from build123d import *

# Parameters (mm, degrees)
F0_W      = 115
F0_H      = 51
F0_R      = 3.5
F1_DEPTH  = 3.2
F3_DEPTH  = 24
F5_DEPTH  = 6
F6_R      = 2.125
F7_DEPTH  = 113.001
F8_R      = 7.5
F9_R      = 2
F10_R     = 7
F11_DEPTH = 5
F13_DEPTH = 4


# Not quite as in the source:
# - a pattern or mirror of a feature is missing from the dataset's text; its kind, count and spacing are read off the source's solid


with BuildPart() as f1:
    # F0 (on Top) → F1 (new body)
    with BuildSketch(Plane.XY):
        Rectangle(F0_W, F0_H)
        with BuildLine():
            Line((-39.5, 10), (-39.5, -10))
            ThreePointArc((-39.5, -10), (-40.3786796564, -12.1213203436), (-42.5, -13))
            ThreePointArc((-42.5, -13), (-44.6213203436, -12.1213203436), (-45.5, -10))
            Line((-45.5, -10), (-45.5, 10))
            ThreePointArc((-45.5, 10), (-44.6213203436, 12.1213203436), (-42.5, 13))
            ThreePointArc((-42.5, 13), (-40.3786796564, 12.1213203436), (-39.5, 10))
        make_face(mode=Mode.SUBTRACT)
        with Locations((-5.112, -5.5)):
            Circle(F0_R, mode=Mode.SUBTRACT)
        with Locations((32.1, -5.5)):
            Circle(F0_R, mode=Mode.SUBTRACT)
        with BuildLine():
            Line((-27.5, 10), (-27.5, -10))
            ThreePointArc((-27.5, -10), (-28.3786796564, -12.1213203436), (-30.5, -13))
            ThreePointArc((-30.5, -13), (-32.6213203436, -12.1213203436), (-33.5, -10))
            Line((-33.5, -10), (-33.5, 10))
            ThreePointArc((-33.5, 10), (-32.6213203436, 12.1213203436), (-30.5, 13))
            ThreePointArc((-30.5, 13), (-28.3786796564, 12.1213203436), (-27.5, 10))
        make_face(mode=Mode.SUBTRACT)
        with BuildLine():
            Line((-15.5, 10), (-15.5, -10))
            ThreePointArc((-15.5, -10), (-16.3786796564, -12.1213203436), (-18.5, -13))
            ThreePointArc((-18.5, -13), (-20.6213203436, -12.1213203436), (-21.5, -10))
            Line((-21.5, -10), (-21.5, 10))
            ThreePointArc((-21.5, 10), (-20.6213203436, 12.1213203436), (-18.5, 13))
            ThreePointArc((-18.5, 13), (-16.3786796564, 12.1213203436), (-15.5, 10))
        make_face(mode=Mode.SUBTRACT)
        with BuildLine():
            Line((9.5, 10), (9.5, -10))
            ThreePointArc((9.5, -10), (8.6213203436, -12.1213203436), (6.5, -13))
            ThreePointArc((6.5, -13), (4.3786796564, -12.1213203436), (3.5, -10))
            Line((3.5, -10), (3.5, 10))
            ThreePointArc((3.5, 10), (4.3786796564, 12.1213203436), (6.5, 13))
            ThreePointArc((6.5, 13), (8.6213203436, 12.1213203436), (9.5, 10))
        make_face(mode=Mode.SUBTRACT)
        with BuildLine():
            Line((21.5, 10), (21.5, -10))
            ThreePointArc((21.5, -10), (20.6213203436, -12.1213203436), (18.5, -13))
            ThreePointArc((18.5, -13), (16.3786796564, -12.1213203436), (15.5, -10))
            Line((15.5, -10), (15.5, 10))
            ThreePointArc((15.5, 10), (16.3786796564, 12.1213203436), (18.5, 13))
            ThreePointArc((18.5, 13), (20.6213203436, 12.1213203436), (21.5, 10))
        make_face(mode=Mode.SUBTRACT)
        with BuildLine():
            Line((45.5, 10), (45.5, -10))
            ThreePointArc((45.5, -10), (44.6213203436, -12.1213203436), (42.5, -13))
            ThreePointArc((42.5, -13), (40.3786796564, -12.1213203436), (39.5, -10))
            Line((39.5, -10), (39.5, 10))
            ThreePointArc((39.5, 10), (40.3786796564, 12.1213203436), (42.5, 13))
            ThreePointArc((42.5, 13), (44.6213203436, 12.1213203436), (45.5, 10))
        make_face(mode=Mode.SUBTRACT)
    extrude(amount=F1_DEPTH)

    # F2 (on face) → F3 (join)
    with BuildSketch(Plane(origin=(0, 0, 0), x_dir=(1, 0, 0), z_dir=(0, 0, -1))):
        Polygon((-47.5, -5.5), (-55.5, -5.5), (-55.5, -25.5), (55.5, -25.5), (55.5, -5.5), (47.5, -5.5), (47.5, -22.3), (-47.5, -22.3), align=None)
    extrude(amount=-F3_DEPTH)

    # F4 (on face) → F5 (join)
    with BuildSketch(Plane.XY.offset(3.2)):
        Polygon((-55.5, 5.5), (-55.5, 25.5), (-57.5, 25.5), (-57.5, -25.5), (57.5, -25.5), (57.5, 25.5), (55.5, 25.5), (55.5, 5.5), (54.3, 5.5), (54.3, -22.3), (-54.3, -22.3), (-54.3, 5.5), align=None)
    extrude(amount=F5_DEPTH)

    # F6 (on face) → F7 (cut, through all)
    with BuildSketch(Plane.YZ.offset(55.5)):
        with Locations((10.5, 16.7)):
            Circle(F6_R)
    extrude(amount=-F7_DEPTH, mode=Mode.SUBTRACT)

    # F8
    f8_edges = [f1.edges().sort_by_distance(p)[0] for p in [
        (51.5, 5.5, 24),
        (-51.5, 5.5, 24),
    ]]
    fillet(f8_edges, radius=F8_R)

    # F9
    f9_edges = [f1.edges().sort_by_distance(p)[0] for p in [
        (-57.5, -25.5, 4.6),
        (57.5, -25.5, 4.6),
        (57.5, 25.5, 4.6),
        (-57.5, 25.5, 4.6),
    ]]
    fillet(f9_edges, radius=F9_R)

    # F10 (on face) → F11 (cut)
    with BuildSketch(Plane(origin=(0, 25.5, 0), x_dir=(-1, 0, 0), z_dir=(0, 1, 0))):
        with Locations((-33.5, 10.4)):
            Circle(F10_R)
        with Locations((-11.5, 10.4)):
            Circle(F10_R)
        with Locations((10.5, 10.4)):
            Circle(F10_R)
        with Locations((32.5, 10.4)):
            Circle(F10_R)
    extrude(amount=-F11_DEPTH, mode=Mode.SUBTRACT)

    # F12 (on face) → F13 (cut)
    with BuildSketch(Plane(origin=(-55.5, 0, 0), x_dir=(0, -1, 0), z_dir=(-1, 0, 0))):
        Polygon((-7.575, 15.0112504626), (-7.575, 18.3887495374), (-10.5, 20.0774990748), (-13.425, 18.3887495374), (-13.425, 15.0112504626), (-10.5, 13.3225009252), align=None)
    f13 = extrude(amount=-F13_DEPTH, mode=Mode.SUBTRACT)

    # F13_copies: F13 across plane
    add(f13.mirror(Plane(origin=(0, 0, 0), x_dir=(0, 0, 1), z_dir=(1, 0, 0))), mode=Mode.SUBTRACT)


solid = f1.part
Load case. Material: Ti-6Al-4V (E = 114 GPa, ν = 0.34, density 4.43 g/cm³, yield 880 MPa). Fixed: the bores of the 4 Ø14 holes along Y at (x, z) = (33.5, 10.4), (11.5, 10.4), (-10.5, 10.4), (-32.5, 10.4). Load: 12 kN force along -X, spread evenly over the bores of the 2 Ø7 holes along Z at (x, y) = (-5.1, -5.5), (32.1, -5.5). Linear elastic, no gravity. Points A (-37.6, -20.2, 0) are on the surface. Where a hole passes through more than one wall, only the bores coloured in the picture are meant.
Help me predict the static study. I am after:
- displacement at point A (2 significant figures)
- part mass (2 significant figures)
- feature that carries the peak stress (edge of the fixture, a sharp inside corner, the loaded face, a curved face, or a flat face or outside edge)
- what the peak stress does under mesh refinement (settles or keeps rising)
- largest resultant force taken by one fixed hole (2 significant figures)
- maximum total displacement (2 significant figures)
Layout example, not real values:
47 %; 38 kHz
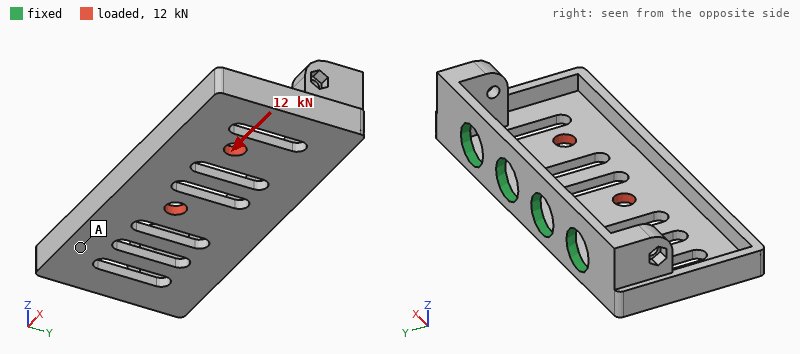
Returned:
0.16 mm; 130 g; edge of the fixture; keeps rising; 5.5 kN; 0.22 mm
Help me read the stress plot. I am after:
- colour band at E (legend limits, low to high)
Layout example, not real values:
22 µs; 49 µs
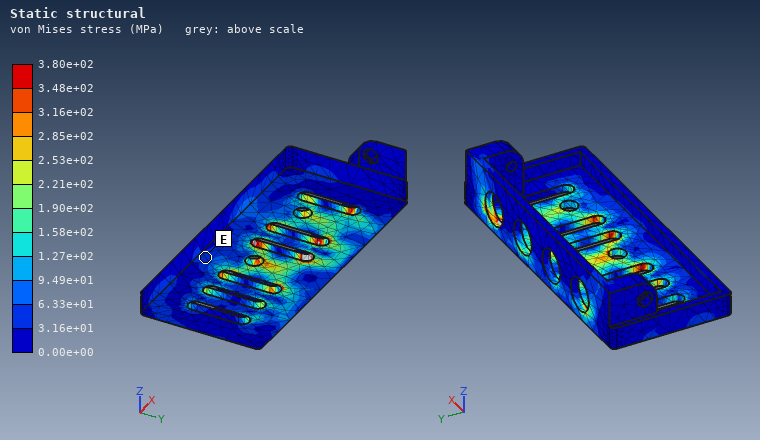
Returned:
3.16e+01 to 6.33e+01 MPa
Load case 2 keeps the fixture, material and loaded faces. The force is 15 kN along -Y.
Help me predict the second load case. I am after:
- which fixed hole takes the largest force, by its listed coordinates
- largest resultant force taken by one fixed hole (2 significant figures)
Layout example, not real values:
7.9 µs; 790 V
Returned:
(33.5, 10.4); 6.3 kN
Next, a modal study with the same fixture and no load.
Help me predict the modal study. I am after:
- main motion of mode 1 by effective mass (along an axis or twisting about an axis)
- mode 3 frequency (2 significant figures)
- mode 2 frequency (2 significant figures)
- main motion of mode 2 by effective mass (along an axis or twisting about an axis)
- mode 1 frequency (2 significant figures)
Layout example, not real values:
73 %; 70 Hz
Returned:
along Z; 4000 Hz; 2200 Hz; twisting about Y; 1300 Hz
